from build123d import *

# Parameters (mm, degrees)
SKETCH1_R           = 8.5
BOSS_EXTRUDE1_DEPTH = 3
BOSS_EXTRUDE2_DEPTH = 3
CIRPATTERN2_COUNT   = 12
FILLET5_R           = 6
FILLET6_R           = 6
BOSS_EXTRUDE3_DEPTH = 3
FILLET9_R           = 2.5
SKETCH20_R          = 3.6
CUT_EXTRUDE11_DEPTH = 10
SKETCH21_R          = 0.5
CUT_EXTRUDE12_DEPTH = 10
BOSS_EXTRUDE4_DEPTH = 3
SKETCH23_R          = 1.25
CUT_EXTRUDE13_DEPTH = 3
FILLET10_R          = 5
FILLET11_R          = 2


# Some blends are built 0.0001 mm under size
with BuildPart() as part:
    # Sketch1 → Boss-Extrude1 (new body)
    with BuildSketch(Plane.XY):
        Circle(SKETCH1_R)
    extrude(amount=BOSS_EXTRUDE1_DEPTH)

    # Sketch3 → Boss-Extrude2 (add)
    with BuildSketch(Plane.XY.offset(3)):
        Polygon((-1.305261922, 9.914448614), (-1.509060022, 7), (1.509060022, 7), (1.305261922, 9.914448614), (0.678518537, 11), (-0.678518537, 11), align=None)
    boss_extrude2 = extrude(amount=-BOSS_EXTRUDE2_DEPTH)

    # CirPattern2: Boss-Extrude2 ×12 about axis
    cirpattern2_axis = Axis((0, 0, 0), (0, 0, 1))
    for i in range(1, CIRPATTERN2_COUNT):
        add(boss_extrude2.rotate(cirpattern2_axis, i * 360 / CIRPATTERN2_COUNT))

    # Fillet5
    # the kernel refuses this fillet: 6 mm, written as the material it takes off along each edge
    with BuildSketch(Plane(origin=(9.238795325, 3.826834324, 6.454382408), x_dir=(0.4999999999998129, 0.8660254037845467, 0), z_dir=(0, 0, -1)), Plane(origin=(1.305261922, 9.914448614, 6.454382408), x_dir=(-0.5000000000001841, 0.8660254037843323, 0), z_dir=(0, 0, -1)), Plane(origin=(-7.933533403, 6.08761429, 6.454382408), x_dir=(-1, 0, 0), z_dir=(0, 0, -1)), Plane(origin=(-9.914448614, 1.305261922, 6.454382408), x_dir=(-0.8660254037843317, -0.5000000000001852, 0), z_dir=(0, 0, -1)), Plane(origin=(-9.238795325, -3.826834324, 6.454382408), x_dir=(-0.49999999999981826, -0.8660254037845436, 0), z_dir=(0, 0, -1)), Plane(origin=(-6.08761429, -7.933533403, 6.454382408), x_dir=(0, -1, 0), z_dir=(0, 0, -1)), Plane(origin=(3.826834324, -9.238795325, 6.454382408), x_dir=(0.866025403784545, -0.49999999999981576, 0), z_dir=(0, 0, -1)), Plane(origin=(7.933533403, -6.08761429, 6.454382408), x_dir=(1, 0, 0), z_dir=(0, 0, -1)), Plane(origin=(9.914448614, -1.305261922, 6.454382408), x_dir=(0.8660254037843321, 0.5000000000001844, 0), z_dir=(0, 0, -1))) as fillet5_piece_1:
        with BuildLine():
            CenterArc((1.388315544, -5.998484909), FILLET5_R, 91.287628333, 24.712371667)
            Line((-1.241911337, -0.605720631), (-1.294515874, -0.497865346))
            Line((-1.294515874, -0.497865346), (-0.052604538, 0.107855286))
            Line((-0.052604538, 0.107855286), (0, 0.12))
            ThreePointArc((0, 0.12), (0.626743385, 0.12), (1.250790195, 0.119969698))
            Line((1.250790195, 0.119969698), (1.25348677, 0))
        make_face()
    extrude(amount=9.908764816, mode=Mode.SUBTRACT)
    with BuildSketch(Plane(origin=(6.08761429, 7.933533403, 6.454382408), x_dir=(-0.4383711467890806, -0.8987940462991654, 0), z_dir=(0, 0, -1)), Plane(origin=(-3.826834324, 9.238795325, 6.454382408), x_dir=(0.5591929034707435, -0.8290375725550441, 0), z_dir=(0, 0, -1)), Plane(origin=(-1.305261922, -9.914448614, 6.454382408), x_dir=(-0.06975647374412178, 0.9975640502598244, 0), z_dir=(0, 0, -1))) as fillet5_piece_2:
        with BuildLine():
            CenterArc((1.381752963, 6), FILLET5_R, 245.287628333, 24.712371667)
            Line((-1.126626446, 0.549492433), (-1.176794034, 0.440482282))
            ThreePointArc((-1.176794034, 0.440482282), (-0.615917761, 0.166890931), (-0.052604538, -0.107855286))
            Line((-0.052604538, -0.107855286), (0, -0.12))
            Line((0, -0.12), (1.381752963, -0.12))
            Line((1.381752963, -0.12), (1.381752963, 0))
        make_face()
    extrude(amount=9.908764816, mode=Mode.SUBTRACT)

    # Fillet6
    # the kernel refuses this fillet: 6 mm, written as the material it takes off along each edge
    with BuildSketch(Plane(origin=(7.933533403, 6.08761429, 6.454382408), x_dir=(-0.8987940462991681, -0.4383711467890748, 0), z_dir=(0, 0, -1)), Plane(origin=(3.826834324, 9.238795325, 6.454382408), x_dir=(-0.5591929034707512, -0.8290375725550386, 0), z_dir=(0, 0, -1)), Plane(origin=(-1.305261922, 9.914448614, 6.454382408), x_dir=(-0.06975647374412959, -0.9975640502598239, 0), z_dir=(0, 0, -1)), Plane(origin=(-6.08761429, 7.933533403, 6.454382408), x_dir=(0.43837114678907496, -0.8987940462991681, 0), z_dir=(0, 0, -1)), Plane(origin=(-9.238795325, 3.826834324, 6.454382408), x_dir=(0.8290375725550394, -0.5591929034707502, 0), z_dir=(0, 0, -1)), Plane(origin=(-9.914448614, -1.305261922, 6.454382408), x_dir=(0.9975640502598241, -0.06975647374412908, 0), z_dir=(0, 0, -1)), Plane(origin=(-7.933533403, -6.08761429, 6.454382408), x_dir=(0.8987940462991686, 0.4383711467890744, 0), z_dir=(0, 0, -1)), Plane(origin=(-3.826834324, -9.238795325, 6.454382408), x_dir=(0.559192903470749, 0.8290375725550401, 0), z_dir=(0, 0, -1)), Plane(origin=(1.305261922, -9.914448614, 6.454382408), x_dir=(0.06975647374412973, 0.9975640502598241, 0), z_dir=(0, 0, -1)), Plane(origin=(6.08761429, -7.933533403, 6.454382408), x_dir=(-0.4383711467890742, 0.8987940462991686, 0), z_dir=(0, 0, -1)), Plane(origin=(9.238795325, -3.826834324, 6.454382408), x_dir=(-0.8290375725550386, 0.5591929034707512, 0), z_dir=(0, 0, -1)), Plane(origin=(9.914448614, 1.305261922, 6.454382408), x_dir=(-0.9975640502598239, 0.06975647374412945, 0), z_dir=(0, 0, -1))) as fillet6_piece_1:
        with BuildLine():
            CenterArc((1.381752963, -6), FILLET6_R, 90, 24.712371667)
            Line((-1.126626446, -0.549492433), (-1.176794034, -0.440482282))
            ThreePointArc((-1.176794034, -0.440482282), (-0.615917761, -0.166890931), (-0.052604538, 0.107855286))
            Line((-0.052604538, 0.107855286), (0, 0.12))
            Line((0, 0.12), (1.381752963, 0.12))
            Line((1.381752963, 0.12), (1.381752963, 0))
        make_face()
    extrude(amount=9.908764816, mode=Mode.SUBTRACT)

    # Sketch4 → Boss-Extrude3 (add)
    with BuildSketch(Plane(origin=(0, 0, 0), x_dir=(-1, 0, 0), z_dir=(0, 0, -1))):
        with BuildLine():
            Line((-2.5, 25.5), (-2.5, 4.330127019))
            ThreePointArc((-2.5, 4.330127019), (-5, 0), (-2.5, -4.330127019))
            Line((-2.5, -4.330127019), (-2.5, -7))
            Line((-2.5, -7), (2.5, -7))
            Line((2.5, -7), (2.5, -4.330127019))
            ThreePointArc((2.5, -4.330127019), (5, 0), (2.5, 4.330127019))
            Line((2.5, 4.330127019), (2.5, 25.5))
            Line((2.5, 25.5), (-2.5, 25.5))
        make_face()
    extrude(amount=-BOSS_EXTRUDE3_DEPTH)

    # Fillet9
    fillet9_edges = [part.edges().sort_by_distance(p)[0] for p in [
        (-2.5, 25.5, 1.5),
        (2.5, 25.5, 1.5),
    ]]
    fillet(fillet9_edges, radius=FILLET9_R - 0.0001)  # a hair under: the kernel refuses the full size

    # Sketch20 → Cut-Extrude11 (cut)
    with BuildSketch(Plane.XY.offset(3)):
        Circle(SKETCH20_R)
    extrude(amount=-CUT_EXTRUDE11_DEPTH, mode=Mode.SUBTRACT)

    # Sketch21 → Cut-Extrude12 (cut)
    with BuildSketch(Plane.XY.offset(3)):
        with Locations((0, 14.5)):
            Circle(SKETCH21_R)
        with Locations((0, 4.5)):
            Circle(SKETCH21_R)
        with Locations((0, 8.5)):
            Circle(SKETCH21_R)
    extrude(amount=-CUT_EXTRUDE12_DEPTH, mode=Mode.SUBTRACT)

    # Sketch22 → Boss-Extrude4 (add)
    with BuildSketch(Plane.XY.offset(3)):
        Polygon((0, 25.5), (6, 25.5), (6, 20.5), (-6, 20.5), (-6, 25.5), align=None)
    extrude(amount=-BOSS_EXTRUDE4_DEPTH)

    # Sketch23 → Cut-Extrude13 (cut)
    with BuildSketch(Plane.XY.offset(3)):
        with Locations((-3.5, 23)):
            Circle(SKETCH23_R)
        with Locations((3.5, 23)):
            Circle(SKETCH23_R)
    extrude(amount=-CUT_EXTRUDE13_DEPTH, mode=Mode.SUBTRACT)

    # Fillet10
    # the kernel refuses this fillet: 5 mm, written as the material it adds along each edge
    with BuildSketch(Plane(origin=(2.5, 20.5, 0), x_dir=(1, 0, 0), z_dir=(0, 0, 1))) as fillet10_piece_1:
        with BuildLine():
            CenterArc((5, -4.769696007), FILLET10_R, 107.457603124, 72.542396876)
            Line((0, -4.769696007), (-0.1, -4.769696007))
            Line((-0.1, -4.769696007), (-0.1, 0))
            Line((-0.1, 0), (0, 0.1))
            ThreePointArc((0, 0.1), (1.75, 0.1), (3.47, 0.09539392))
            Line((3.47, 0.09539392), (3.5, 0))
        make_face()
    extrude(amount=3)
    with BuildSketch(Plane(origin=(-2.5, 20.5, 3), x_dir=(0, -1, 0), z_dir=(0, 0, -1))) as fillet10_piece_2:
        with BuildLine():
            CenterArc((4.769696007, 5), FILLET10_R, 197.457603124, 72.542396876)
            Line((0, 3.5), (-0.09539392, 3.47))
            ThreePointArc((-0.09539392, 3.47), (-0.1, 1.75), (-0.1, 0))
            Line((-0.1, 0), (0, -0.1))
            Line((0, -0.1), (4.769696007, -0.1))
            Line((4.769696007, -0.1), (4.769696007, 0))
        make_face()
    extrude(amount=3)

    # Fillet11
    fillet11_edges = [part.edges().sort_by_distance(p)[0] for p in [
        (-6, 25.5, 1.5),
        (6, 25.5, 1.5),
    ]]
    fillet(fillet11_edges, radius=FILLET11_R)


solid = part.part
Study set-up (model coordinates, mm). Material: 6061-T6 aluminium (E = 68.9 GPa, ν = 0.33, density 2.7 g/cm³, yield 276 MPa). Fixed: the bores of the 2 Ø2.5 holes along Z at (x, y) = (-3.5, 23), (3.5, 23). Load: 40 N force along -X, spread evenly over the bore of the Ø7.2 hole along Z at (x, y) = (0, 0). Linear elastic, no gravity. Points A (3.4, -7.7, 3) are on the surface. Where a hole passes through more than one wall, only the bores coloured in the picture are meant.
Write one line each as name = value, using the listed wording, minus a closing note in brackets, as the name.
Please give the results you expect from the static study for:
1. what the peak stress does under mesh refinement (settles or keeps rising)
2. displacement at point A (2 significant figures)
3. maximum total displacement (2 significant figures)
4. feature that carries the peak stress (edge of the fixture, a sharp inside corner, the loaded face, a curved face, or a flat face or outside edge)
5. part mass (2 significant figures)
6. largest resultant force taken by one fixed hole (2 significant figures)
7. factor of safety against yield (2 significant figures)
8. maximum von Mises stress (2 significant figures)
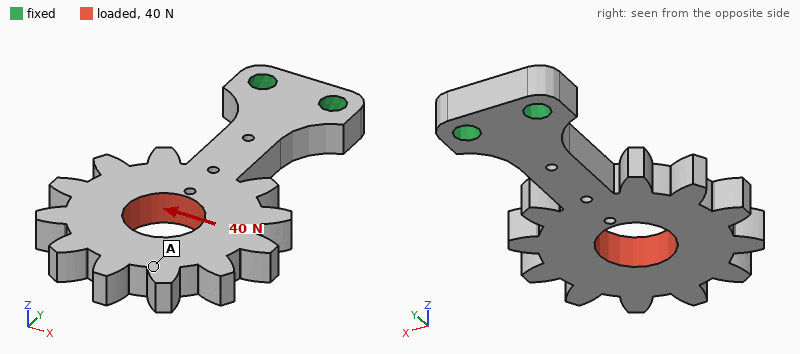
what the peak stress does under mesh refinement = settles
displacement at point A = 69 µm
maximum total displacement = 79 µm
feature that carries the peak stress = a curved face
part mass = 3.0 g
largest resultant force taken by one fixed hole = 120 N
factor of safety against yield = 4.8
maximum von Mises stress = 57 MPa
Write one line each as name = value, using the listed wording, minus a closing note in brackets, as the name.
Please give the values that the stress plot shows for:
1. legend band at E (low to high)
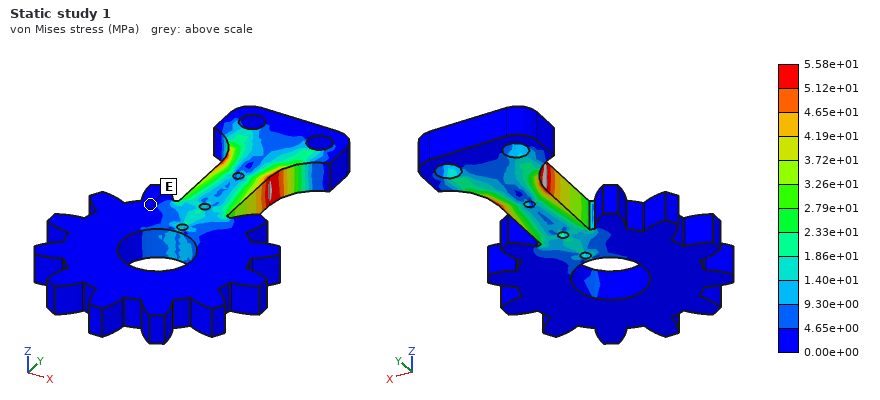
legend band at E = 0.00e+00 to 4.65e+00 MPa
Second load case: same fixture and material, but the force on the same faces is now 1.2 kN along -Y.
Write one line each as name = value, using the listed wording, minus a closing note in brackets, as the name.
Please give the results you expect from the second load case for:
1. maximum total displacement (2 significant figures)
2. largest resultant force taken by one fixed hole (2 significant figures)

maximum total displacement = 31 µm
largest resultant force taken by one fixed hole = 640 N
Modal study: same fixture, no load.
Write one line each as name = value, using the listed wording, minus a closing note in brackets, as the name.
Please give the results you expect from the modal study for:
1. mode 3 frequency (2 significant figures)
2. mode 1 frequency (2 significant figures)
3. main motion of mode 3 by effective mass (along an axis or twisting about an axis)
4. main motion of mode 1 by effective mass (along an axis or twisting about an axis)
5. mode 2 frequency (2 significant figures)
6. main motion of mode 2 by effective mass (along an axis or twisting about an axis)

mode 3 frequency = 4500 Hz
mode 1 frequency = 1600 Hz
main motion of mode 3 by effective mass = twisting about Y
main motion of mode 1 by effective mass = along Z
mode 2 frequency = 2900 Hz
main motion of mode 2 by effective mass = along X
